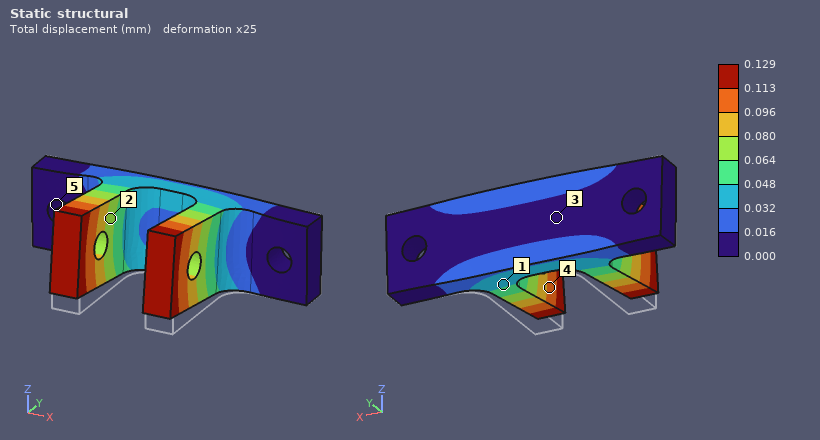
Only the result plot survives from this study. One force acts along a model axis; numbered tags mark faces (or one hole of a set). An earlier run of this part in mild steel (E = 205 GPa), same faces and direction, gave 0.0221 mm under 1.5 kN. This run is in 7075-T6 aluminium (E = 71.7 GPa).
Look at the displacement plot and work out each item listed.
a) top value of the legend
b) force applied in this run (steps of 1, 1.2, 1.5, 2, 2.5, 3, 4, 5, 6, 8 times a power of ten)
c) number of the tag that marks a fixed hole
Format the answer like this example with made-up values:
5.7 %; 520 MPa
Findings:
0.129 mm; 3 kN; 5
